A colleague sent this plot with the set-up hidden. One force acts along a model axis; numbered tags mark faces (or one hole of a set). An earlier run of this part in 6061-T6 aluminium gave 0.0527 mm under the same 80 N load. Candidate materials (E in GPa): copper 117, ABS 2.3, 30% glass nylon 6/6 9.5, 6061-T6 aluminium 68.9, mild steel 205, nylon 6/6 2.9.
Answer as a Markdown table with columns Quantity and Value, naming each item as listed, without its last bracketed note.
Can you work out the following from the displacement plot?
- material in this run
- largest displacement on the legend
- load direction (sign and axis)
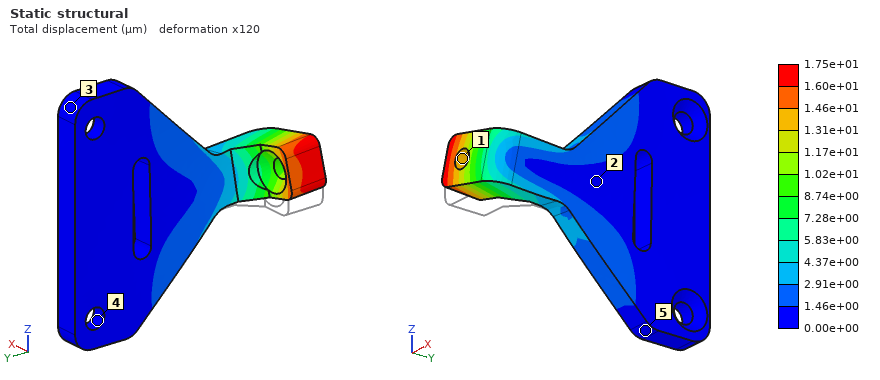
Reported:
| Quantity | Value |
|---|---|
| material in this run | mild steel |
| largest displacement on the legend | 1.75e+01 µm |
| load direction | +Z |
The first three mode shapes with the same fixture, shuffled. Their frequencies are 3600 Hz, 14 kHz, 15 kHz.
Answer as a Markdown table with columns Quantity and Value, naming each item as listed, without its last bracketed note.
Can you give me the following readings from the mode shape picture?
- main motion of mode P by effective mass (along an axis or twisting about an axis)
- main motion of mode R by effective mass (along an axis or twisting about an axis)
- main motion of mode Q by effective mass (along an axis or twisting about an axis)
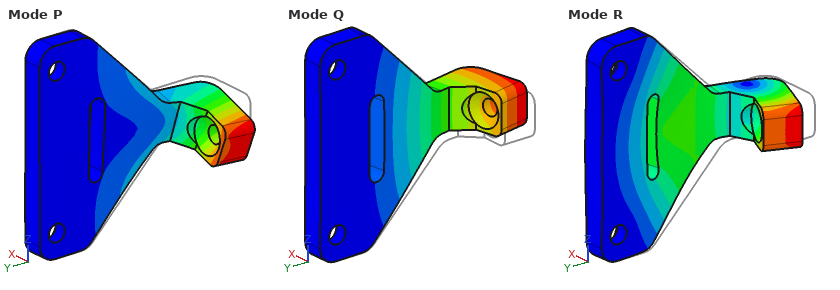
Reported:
| Quantity | Value |
|---|---|
| main motion of mode P by effective mass | along Z |
| main motion of mode R by effective mass | along X |
| main motion of mode Q by effective mass | along X |
